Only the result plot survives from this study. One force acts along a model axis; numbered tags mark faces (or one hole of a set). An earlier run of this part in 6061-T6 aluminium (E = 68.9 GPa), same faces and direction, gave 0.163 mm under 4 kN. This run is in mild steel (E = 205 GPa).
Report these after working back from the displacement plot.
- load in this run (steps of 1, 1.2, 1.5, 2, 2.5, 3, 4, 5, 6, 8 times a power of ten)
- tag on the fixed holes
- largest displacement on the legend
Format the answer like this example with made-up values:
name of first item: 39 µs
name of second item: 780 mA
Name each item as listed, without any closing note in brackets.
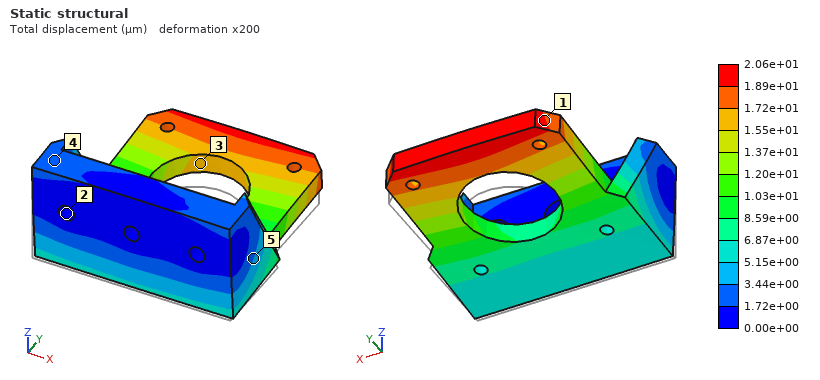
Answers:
load in this run: 1.5 kN
tag on the fixed holes: 2
largest displacement on the legend: 2.06e+01 µm
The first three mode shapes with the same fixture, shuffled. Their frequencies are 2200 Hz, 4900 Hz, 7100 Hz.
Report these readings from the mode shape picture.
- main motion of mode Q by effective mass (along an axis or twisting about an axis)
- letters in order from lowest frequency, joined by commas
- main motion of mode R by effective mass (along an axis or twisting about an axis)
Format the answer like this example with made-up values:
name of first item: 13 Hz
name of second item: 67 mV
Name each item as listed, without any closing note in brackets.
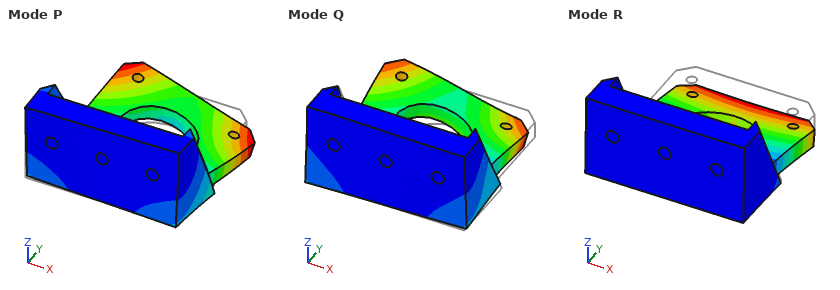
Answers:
main motion of mode Q by effective mass: along X
letters in order from lowest frequency, joined by commas: R, P, Q
main motion of mode R by effective mass: along Z
